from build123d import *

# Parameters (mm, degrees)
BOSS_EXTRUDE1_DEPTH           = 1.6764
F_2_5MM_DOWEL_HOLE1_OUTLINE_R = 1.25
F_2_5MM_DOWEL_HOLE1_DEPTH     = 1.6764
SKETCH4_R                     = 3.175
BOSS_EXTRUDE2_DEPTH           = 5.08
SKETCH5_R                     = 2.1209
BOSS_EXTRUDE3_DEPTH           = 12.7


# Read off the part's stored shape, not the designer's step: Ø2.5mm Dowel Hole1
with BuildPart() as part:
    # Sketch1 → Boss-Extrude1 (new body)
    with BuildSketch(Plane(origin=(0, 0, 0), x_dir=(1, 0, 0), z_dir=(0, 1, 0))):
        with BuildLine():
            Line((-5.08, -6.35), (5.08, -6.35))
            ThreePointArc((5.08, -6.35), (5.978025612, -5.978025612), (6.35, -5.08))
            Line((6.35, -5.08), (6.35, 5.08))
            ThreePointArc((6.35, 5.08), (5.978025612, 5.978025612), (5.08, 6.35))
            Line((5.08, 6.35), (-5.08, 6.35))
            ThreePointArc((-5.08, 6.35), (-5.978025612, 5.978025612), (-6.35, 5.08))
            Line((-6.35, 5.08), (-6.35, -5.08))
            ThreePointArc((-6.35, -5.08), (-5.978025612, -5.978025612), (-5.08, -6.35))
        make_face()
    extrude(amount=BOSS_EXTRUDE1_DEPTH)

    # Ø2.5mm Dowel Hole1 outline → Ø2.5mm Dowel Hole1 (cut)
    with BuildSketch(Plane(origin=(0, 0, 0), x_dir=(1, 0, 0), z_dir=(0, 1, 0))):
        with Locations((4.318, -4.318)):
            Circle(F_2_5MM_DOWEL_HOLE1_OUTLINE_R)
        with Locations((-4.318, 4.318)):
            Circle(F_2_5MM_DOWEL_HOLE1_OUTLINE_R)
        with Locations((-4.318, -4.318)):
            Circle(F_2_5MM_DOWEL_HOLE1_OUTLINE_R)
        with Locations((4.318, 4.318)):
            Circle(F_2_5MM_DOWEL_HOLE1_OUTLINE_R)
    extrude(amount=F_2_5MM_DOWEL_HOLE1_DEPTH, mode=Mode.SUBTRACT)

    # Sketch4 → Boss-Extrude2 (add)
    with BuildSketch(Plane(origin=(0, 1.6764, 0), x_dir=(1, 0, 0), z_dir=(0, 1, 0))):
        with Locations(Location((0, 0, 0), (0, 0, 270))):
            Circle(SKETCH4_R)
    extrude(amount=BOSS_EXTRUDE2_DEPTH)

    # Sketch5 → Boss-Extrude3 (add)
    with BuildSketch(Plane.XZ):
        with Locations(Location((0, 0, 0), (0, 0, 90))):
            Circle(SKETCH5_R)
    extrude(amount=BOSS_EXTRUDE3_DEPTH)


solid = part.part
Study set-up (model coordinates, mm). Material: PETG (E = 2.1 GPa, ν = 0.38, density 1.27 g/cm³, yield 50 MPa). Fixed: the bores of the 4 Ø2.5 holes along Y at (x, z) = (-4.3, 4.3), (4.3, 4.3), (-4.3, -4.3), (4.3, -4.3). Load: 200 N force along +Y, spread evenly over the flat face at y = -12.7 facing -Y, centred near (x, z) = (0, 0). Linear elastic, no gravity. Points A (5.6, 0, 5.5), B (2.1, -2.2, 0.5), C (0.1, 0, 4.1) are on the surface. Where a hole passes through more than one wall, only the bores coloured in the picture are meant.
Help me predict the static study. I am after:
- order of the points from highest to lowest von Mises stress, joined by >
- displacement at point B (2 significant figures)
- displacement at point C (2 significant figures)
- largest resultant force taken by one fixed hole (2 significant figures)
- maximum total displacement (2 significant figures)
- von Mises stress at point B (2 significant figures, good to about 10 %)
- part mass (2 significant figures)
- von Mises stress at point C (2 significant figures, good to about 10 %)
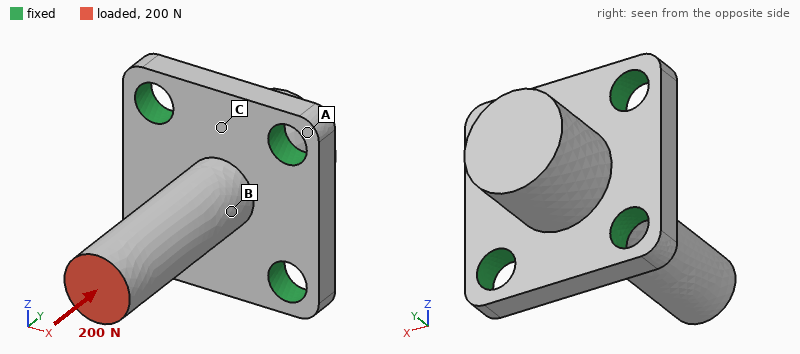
B > C > A
0.070 mm
0.029 mm
50 N
0.14 mm
14 MPa
0.73 g
8.3 MPa
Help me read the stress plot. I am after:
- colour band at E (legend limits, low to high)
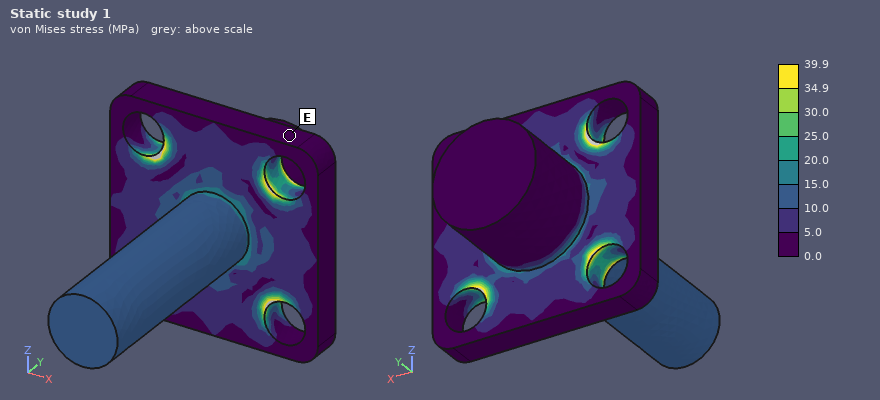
0.0 to 5.0 MPa
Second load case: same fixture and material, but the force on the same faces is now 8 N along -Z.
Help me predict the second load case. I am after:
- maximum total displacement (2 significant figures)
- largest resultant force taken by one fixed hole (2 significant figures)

0.25 mm
8.2 N
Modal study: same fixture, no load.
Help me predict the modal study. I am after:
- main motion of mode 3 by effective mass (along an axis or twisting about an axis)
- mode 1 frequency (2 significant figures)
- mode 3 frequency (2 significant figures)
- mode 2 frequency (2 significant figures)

along Y
3600 Hz
13 kHz
3600 Hz
